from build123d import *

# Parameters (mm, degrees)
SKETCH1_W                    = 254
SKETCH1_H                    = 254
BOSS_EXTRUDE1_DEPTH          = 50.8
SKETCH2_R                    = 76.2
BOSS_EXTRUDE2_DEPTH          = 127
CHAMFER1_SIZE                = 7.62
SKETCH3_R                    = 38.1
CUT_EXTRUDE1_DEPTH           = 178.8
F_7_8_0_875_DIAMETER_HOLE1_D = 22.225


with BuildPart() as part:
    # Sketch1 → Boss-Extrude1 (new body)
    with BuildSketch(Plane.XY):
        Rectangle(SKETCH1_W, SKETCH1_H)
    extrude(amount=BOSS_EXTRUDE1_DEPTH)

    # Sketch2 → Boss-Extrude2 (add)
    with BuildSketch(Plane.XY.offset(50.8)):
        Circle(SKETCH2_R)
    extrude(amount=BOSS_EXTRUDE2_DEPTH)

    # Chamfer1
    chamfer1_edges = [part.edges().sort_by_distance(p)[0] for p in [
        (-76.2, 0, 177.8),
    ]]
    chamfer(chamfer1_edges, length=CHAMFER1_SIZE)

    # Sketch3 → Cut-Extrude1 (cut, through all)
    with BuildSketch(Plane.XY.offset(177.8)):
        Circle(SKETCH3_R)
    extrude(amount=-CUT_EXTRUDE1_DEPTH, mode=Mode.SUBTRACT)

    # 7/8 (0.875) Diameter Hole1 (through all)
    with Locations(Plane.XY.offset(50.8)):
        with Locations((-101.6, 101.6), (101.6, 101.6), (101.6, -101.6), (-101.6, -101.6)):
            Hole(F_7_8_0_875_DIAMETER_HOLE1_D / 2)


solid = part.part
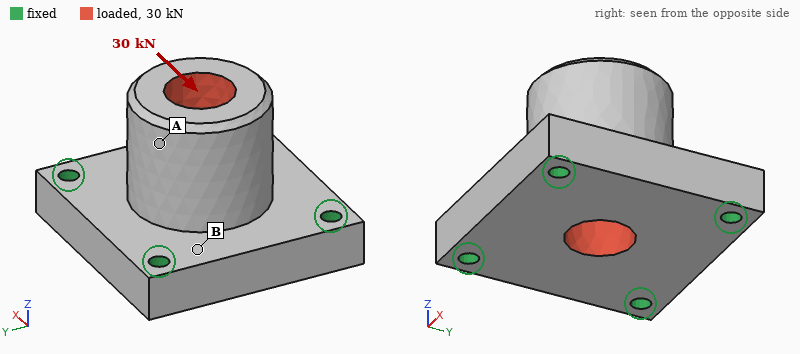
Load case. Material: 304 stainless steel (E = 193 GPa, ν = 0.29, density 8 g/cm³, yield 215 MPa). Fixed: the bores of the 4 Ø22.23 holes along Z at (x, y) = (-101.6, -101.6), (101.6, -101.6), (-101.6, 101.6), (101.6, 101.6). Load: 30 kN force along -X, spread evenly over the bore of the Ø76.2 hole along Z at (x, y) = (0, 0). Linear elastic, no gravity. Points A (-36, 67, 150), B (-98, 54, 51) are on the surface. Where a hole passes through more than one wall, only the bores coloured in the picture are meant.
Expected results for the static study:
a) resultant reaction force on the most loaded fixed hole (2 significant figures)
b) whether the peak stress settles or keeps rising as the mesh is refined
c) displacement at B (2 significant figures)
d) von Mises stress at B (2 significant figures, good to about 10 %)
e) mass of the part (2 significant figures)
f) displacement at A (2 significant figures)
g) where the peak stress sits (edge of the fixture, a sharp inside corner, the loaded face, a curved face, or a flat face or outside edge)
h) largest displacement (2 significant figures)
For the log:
9.8 kN
keeps rising
1.7 µm
2.6 MPa
38 kg
8.2 µm
edge of the fixture
10 µm
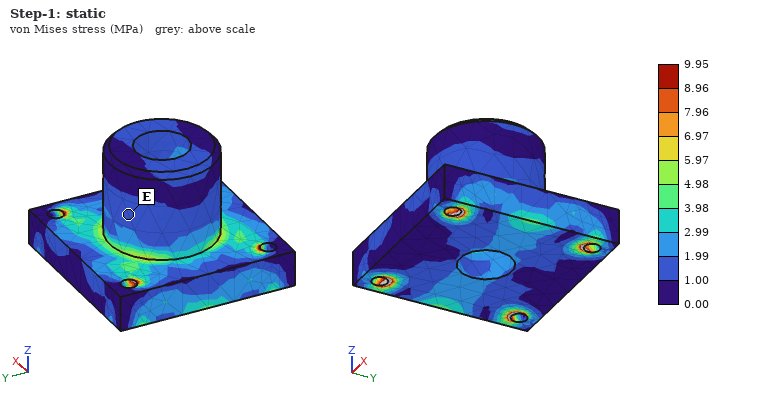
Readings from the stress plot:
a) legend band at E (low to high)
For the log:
1.00 to 1.99 MPa
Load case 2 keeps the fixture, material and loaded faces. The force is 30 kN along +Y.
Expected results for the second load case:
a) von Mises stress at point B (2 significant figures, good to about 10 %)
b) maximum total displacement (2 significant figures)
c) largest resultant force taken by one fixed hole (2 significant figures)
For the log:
3.5 MPa
10 µm
9.8 kN
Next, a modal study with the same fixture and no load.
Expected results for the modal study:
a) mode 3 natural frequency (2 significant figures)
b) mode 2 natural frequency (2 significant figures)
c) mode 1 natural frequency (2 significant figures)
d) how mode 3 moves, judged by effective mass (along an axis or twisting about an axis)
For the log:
2600 Hz
2200 Hz
2200 Hz
along Z
